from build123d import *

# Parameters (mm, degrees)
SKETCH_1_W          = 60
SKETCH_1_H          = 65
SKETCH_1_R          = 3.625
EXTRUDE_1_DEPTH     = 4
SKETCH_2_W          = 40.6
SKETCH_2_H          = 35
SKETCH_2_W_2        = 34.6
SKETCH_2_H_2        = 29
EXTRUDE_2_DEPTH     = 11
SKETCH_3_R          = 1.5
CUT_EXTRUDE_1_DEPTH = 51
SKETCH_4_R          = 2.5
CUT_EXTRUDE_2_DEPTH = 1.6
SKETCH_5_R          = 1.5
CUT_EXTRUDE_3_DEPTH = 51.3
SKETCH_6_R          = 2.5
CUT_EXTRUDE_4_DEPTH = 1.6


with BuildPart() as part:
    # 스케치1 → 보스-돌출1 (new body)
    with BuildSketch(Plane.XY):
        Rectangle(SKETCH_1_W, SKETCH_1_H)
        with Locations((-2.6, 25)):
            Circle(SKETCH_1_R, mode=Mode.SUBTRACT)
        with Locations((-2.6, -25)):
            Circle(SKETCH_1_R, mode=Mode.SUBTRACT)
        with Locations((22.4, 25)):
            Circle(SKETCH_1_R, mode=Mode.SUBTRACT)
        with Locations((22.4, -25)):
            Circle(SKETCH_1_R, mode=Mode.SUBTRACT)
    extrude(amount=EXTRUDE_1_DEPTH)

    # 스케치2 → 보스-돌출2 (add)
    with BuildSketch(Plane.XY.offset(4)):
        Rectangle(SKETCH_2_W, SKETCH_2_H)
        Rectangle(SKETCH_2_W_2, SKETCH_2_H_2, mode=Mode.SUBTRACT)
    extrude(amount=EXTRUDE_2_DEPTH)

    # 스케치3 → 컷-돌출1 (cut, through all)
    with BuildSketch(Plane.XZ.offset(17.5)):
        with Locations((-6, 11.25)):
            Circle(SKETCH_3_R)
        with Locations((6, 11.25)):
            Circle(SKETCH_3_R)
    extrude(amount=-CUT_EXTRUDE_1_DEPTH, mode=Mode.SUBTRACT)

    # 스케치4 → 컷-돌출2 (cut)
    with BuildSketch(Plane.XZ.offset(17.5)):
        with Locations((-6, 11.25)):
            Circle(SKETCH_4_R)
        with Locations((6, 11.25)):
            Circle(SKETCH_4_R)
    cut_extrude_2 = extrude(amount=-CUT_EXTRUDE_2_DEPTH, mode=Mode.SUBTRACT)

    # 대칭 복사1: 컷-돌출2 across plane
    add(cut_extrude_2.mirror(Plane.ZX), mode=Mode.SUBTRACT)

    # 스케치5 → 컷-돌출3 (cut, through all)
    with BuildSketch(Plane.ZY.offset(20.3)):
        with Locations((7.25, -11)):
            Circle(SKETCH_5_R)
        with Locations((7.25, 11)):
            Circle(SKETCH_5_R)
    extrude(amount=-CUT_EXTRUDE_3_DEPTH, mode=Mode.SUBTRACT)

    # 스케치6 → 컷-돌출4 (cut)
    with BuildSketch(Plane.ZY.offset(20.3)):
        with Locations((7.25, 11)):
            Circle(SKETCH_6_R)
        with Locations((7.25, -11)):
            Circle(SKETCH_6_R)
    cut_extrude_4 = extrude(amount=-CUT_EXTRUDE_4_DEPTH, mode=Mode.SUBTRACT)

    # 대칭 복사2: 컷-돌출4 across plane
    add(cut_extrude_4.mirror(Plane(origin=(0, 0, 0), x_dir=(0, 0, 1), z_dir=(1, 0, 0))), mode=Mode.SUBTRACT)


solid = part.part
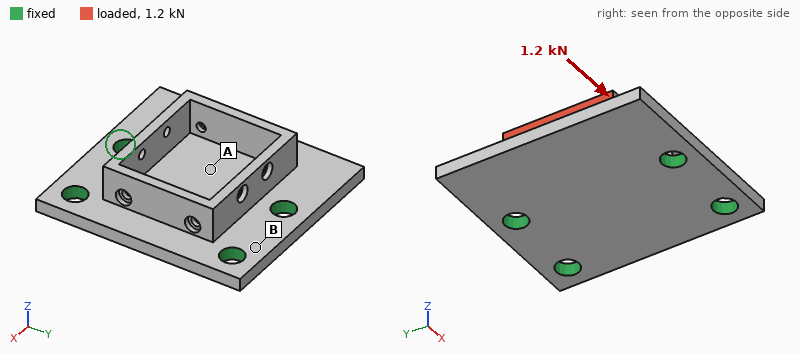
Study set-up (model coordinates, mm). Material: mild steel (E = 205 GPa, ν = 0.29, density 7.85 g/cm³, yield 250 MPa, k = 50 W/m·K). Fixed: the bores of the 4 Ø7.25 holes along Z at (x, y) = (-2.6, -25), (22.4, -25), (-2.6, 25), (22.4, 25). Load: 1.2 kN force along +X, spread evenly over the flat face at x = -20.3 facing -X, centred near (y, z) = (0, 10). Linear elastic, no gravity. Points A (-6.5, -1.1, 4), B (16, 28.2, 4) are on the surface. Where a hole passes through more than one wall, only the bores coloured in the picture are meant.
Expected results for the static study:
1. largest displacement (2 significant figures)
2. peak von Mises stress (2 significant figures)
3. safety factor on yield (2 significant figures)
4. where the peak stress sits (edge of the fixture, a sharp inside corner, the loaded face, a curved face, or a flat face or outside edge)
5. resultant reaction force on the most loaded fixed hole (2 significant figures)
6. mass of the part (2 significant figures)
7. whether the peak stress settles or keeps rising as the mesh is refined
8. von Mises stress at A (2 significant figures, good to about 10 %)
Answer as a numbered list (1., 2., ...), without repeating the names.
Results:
1. 20 µm
2. 83 MPa
3. 3.0
4. a curved face
5. 390 N
6. 150 g
7. settles
8. 11 MPa
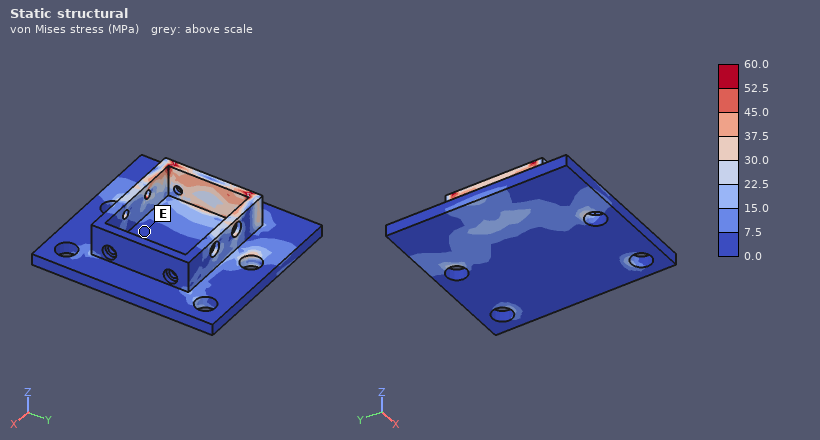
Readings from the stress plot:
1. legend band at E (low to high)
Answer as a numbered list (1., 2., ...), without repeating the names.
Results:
1. 0.0 to 7.5 MPa
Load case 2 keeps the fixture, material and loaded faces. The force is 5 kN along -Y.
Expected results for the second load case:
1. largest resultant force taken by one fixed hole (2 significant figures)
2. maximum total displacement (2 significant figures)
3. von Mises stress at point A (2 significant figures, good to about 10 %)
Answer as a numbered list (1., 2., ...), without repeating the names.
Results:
1. 3.1 kN
2. 25 µm
3. 42 MPa
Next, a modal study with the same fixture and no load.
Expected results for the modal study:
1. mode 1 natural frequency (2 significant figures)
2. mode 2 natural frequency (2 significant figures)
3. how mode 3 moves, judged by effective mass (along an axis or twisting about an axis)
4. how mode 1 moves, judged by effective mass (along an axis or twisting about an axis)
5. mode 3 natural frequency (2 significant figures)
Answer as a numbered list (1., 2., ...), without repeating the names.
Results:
1. 5900 Hz
2. 8200 Hz
3. along Z
4. along Z
5. 11 kHz
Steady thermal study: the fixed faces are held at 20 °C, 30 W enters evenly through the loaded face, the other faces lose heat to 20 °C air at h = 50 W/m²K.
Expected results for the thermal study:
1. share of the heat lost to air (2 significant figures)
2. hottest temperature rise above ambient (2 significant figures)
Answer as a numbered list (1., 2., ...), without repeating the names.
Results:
1. 28 %
2. 72 K
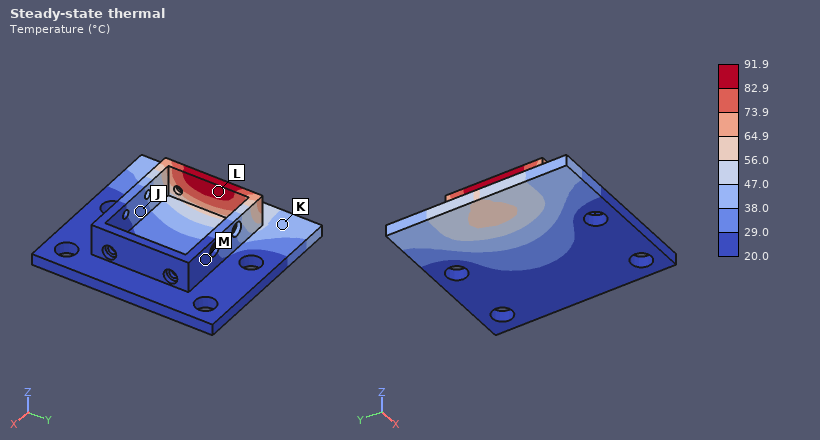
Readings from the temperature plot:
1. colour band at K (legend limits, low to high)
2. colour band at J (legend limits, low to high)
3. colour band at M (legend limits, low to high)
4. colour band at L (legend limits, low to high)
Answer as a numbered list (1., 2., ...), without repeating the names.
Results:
1. 38.0 to 47.0 °C
2. 29.0 to 38.0 °C
3. 20.0 to 29.0 °C
4. 82.9 to 91.9 °C
